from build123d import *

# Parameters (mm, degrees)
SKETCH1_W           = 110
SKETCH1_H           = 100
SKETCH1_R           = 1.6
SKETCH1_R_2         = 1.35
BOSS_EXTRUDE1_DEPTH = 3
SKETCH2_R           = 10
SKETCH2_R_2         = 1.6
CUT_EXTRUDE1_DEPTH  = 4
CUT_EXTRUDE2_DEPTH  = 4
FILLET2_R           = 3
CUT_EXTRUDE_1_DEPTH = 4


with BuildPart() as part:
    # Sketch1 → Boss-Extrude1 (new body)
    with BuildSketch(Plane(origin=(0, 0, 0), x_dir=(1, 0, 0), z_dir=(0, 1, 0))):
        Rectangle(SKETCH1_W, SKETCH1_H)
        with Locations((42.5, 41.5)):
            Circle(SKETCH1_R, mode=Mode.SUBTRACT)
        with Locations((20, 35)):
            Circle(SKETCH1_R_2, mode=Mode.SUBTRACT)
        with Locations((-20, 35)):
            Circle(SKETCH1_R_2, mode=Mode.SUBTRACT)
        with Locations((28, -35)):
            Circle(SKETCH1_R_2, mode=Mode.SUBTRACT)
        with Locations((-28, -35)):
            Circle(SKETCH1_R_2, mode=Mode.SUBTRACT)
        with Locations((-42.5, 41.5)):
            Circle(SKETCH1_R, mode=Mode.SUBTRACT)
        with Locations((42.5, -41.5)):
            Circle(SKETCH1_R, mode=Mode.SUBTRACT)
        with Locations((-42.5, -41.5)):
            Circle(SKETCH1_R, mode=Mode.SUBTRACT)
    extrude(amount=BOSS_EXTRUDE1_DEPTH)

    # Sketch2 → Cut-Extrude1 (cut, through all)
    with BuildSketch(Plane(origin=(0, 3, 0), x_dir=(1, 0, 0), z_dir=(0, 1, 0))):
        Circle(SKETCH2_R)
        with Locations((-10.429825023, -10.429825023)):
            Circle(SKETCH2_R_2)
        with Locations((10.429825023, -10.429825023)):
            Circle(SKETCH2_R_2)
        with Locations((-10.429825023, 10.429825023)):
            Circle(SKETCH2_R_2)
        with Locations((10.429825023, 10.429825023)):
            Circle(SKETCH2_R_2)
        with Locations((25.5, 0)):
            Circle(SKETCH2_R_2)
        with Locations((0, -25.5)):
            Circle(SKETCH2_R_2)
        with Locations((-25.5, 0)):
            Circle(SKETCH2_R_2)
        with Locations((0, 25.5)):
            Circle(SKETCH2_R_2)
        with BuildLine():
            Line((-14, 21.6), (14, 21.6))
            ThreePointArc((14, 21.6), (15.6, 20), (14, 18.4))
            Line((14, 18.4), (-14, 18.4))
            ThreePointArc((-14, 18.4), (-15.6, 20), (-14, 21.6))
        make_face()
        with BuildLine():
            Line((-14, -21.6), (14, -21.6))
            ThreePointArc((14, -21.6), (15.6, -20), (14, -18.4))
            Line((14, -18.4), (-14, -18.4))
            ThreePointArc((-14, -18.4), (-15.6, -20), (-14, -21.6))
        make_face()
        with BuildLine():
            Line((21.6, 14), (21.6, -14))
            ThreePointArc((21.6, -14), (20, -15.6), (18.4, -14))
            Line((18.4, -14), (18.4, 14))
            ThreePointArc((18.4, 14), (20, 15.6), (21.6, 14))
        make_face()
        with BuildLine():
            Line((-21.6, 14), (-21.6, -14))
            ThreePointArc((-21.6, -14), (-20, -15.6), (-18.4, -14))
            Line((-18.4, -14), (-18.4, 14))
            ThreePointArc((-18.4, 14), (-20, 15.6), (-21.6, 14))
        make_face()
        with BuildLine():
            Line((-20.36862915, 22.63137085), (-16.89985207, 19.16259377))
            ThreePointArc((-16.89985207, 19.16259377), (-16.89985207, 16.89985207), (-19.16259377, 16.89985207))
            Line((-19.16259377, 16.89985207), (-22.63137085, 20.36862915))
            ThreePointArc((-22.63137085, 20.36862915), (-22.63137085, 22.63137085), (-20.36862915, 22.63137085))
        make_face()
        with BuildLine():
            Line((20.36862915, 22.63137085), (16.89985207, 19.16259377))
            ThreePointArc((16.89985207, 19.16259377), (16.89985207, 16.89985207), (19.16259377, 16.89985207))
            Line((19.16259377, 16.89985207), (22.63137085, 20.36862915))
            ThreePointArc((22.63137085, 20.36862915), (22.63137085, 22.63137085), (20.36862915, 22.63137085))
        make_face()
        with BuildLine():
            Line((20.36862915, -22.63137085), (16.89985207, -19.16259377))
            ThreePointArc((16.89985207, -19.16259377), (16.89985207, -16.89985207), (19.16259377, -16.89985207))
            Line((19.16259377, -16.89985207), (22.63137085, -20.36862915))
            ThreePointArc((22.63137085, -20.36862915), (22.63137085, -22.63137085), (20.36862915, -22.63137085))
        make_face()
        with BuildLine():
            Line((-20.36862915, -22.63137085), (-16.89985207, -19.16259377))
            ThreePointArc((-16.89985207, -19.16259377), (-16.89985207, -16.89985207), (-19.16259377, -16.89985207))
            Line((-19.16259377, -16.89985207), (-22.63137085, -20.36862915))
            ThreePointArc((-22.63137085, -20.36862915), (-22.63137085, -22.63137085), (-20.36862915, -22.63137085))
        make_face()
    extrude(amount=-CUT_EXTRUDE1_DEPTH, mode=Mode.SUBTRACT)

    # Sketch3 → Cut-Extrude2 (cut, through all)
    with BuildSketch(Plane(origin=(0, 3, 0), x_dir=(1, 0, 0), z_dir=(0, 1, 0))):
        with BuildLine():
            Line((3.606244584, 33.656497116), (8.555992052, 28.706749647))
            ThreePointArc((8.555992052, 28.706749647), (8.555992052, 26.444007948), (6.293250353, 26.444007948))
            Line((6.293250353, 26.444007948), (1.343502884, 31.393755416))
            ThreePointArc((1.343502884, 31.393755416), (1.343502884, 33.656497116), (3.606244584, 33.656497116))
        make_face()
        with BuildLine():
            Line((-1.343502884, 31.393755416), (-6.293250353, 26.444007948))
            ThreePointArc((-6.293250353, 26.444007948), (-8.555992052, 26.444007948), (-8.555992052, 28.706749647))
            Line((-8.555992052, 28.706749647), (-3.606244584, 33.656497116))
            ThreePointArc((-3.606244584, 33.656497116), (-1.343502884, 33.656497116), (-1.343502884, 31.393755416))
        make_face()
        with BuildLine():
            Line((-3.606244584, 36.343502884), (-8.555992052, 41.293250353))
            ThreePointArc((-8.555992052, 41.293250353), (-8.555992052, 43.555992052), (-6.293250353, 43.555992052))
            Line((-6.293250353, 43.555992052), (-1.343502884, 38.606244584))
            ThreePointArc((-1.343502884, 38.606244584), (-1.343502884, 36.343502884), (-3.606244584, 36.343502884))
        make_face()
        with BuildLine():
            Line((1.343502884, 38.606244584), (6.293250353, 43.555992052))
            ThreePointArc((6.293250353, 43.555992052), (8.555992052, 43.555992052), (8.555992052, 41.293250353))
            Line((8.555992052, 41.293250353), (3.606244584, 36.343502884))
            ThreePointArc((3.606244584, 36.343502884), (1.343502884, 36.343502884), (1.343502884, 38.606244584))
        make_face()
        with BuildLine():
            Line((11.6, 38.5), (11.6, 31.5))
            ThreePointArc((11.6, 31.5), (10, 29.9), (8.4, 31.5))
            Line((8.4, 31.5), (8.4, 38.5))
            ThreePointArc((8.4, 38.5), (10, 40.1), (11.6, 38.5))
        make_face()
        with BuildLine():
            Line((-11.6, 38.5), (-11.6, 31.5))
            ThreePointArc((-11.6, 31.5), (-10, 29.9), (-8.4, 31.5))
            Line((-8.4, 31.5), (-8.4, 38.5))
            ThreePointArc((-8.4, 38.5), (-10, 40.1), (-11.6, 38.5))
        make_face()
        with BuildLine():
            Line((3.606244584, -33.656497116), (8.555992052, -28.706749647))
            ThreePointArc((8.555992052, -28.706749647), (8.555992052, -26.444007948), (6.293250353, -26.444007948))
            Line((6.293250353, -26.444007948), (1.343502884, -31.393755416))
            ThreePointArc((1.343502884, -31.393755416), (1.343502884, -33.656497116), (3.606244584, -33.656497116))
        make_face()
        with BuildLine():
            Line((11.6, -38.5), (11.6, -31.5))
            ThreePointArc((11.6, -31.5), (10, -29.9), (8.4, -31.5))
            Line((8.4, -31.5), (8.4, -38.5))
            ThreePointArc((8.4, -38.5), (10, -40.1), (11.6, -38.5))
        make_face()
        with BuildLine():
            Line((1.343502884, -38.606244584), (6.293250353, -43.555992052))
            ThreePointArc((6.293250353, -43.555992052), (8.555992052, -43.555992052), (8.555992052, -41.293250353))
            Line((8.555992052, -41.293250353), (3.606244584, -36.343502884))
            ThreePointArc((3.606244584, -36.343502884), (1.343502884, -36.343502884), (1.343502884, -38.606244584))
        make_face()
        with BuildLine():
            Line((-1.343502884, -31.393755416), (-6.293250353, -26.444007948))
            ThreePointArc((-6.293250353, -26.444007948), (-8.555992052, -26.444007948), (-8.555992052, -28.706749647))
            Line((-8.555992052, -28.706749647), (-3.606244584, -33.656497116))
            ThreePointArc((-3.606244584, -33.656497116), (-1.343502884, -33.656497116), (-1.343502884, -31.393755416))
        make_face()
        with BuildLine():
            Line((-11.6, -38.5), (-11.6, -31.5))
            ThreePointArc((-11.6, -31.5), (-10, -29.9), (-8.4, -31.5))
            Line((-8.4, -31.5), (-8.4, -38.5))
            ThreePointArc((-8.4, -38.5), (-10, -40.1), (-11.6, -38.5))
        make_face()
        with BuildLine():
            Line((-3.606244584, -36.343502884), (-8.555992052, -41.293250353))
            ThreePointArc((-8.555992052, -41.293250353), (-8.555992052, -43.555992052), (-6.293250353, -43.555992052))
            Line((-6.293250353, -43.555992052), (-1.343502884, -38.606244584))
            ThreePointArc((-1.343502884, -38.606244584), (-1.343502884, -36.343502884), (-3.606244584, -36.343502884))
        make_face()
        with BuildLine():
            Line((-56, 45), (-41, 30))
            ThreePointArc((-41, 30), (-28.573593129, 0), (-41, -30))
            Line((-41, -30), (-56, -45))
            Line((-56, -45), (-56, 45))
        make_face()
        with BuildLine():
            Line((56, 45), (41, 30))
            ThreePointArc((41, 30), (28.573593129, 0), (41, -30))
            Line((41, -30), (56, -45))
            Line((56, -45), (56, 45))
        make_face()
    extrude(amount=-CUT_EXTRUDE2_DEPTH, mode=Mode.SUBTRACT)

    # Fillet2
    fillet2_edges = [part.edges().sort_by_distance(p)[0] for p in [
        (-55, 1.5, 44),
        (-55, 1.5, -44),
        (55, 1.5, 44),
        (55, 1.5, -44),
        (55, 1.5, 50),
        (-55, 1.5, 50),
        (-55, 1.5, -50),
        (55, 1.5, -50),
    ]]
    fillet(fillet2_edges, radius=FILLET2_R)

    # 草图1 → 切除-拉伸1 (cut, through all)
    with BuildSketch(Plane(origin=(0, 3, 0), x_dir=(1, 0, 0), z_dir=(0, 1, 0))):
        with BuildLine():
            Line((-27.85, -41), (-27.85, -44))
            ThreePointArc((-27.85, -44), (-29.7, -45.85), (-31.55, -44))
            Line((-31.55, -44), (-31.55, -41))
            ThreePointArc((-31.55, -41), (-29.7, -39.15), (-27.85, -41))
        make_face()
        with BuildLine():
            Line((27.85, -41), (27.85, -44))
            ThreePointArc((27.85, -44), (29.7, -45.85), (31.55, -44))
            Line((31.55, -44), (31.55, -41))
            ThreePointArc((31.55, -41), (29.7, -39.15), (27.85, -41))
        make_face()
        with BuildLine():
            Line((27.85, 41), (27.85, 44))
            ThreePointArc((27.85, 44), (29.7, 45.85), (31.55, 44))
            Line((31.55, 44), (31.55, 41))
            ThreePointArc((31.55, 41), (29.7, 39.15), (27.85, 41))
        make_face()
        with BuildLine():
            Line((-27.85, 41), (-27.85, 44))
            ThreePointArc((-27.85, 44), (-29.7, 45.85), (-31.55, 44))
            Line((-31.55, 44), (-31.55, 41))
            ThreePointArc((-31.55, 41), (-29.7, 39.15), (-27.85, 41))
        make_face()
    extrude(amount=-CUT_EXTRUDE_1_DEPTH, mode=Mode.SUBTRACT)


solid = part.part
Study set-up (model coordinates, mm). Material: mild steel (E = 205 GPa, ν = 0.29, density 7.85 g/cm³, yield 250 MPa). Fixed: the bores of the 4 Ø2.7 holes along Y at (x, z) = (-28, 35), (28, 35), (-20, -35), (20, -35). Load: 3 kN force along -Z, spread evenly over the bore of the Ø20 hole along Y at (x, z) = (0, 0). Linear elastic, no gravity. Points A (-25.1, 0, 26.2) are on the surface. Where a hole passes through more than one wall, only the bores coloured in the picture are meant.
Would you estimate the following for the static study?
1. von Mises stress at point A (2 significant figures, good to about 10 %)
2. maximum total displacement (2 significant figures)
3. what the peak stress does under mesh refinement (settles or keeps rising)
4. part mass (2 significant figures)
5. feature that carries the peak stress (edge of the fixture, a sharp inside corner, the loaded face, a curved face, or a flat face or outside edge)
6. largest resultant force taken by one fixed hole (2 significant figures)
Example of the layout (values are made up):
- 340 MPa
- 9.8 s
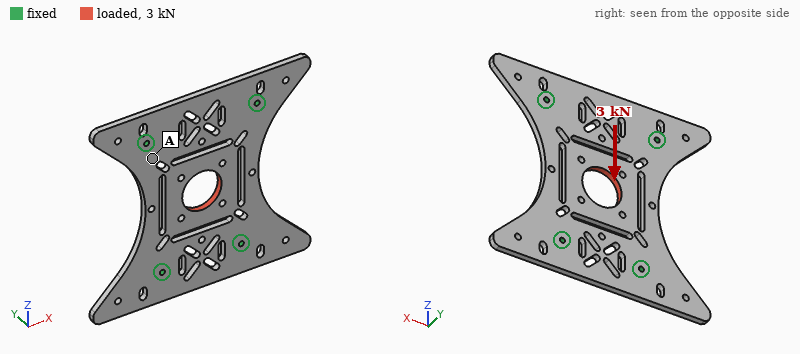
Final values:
- 16 MPa
- 10.0 µm
- keeps rising
- 150 g
- a sharp inside corner
- 800 N
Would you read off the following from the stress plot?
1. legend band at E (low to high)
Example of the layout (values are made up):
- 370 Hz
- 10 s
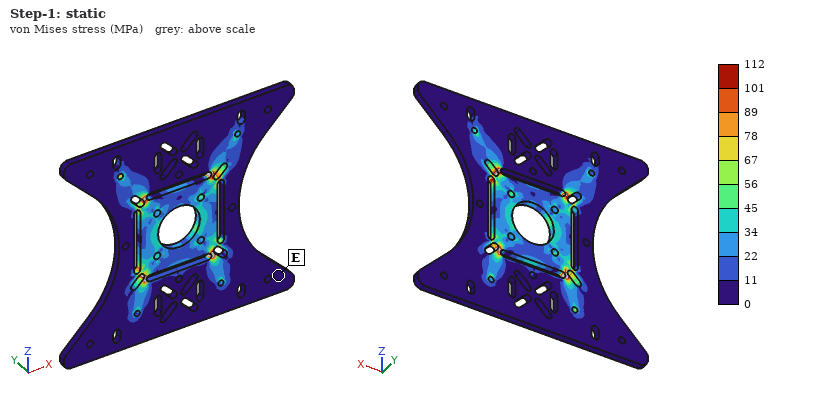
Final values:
- 0 to 11 MPa
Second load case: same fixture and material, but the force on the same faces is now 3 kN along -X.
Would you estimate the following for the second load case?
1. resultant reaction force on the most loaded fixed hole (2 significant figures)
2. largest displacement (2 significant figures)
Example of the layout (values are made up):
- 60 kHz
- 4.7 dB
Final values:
- 1.0 kN
- 14 µm
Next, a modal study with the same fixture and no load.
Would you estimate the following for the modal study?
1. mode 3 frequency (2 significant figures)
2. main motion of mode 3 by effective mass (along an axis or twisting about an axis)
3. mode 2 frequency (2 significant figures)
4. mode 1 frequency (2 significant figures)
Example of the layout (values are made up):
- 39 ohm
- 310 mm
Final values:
- 2700 Hz
- along Y
- 2500 Hz
- 2400 Hz
